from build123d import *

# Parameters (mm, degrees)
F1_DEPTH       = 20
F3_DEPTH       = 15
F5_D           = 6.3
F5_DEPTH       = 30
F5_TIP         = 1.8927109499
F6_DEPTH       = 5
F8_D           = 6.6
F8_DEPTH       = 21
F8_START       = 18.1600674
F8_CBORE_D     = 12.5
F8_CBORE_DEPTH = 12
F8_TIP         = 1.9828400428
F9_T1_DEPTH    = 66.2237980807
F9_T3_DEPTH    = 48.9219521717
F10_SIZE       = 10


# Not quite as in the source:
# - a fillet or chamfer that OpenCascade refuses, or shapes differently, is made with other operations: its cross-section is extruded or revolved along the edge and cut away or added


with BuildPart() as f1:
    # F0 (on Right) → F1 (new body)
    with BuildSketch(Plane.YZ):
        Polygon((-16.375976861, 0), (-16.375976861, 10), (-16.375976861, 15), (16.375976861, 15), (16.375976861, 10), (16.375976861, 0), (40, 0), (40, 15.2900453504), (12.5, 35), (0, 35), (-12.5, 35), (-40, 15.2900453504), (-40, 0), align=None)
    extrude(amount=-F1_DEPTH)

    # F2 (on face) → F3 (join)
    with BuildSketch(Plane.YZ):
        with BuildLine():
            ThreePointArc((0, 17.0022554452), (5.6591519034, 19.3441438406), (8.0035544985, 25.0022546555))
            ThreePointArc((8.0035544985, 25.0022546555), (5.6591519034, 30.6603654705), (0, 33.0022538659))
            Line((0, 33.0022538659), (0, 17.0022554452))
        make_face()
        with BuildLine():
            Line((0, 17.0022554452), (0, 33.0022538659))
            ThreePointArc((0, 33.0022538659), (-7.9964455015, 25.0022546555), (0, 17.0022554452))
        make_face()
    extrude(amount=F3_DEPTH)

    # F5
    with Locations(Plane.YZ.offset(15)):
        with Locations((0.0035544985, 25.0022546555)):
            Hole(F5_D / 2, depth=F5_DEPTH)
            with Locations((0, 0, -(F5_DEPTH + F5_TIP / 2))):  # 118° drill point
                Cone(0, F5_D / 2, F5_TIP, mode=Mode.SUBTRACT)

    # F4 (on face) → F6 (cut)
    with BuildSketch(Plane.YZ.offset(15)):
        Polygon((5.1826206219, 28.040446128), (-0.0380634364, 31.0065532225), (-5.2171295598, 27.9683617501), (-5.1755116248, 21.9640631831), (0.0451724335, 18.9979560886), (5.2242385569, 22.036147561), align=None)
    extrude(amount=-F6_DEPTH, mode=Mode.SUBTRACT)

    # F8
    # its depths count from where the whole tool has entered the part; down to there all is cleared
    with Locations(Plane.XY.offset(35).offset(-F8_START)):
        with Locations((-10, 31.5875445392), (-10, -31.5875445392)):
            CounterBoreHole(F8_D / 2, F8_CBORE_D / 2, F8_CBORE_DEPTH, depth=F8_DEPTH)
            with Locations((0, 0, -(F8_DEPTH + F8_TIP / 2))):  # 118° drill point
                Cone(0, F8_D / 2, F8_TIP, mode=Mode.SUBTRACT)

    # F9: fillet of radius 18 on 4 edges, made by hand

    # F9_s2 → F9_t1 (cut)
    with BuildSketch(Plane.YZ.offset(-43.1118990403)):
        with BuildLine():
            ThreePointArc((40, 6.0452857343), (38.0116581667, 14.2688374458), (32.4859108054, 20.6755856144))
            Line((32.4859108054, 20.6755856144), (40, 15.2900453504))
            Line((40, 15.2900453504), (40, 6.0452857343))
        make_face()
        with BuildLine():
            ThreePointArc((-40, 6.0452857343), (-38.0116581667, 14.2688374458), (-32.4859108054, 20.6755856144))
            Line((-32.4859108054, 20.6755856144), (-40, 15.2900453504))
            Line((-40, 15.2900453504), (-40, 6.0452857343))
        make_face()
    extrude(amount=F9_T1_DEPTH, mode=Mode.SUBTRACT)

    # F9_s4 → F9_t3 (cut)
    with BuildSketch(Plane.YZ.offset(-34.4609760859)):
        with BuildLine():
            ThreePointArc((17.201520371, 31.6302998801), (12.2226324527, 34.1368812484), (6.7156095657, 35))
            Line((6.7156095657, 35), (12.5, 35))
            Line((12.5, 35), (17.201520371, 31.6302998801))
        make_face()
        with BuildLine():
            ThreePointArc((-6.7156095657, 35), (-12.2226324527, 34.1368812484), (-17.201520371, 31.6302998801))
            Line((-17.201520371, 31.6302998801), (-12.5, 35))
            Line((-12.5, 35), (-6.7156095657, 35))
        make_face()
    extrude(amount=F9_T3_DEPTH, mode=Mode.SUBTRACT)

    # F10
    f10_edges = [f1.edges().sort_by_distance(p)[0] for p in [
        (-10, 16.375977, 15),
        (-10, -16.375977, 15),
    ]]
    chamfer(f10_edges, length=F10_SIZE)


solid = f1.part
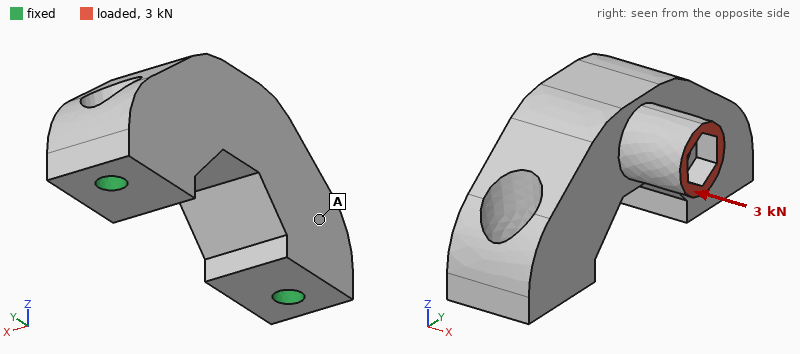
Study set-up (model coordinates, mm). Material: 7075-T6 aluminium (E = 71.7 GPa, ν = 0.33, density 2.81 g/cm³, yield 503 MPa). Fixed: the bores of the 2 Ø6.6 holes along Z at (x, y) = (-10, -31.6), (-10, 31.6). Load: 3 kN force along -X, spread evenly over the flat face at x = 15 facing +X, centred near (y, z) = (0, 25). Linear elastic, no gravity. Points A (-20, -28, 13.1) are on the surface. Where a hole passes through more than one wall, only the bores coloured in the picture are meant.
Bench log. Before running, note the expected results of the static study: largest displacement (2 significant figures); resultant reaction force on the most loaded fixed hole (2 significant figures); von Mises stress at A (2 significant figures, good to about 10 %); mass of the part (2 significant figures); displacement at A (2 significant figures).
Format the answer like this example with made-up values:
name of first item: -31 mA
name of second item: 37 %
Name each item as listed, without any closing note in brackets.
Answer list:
largest displacement: 0.16 mm
resultant reaction force on the most loaded fixed hole: 1.5 kN
von Mises stress at A: 34 MPa
mass of the part: 96 g
displacement at A: 0.054 mm
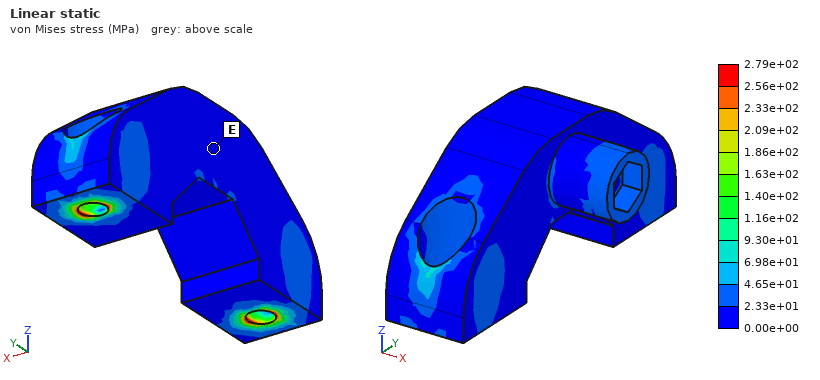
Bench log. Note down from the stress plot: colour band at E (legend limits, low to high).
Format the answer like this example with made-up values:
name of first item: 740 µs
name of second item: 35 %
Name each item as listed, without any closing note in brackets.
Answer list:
colour band at E: 0.00e+00 to 2.33e+01 MPa
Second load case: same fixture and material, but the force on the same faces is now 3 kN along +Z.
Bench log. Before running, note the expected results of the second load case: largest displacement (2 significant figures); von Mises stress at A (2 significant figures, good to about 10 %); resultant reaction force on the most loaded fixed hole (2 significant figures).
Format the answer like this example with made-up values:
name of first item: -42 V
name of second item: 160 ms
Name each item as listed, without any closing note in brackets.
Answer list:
largest displacement: 0.25 mm
von Mises stress at A: 40 MPa
resultant reaction force on the most loaded fixed hole: 2.1 kN
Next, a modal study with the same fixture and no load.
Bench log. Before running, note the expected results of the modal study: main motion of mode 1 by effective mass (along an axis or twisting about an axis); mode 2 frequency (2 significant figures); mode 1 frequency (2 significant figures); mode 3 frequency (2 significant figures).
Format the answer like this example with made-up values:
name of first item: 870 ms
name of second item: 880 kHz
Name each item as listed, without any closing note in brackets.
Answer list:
main motion of mode 1 by effective mass: along X
mode 2 frequency: 12 kHz
mode 1 frequency: 3500 Hz
mode 3 frequency: 12 kHz
